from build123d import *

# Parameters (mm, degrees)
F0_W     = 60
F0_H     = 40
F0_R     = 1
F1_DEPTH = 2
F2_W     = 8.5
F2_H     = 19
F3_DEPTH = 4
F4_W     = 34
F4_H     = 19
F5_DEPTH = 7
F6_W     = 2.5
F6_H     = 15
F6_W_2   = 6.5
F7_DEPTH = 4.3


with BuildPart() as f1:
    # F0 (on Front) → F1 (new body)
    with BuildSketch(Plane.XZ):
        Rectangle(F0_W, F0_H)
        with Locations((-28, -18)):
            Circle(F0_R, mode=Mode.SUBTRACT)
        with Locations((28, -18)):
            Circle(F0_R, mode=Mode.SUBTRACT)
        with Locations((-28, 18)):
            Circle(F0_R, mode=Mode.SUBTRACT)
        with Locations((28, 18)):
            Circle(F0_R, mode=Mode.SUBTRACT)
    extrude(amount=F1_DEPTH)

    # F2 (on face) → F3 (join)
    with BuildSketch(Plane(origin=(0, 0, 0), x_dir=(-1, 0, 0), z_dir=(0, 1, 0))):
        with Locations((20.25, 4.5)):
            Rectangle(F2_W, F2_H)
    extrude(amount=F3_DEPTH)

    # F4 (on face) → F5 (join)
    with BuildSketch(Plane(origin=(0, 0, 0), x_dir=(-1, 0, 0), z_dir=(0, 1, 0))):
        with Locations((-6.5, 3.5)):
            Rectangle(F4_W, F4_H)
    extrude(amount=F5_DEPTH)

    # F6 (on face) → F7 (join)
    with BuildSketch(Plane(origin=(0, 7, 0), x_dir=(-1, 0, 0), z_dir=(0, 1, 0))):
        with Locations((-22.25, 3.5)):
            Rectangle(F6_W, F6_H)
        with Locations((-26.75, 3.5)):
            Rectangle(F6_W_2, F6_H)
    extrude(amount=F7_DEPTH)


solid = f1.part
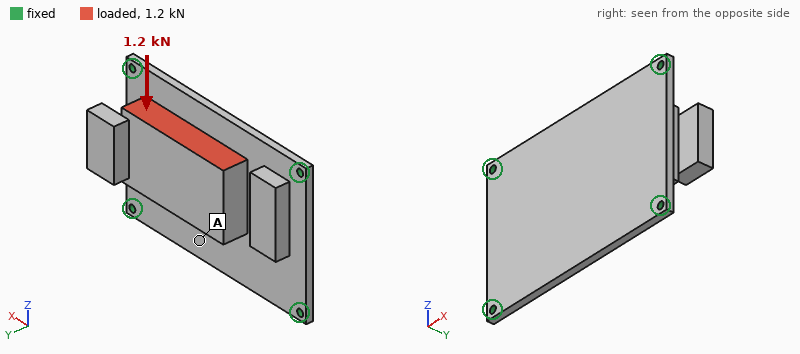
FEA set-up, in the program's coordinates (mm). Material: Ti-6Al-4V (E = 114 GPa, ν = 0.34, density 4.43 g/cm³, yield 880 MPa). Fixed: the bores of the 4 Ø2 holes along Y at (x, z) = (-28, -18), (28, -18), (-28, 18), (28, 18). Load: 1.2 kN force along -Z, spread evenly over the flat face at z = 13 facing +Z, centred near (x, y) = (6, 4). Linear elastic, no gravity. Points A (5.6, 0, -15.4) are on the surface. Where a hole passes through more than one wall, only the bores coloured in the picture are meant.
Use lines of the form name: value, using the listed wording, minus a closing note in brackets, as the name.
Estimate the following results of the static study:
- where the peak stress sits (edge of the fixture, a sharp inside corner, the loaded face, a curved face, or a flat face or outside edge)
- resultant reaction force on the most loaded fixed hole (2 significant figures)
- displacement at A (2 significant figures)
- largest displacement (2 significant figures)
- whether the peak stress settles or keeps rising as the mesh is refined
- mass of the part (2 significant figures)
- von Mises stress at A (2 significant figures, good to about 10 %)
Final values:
where the peak stress sits: edge of the fixture
resultant reaction force on the most loaded fixed hole: 460 N
displacement at A: 30 µm
largest displacement: 34 µm
whether the peak stress settles or keeps rising as the mesh is refined: keeps rising
mass of the part: 47 g
von Mises stress at A: 13 MPa
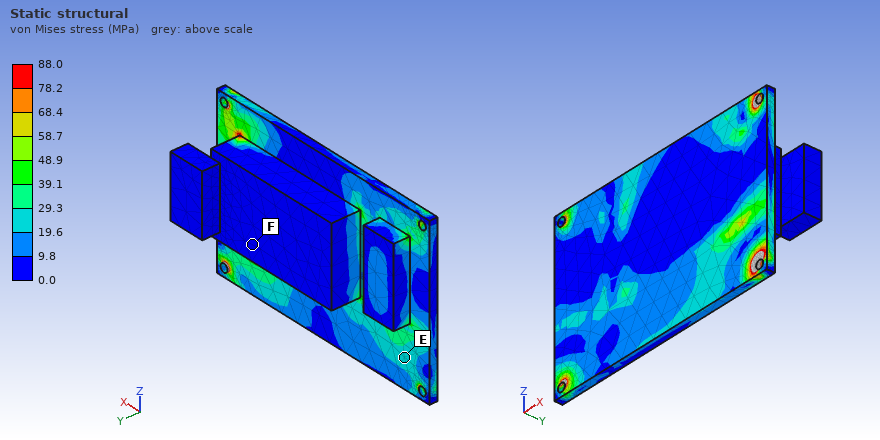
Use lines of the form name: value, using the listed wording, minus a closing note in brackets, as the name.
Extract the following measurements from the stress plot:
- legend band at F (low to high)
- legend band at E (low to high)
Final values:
legend band at F: 0.0 to 9.8 MPa
legend band at E: 19.6 to 29.3 MPa
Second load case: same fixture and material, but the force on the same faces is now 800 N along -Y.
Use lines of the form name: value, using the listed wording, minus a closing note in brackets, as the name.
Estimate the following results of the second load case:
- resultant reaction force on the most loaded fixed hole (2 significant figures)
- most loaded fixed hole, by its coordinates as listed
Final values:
resultant reaction force on the most loaded fixed hole: 520 N
most loaded fixed hole, by its coordinates as listed: (28, 18)
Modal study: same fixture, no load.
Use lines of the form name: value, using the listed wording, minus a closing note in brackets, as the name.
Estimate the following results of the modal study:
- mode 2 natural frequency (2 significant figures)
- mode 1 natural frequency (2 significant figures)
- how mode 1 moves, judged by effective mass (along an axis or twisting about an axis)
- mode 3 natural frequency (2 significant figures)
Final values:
mode 2 natural frequency: 4900 Hz
mode 1 natural frequency: 2600 Hz
how mode 1 moves, judged by effective mass: along Y
mode 3 natural frequency: 6100 Hz
